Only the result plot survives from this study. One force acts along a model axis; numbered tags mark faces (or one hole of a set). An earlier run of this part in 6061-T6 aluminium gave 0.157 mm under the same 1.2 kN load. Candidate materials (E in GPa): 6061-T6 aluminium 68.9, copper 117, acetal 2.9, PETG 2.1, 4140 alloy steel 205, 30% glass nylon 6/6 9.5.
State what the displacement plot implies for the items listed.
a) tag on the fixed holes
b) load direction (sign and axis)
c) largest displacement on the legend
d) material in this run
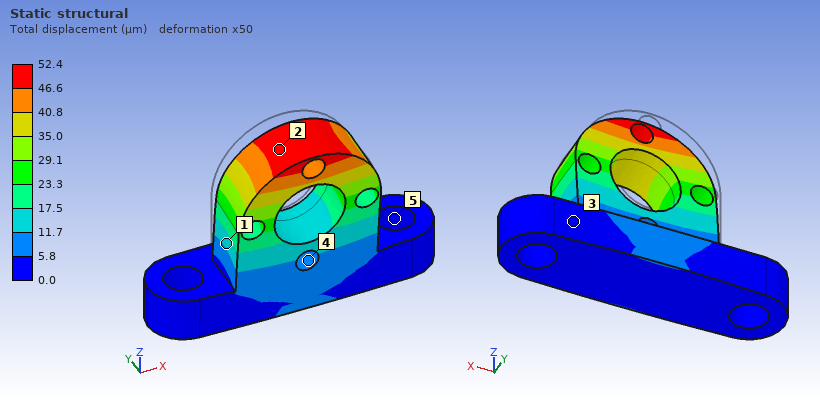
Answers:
5
-Y
52.4 µm
4140 alloy steel
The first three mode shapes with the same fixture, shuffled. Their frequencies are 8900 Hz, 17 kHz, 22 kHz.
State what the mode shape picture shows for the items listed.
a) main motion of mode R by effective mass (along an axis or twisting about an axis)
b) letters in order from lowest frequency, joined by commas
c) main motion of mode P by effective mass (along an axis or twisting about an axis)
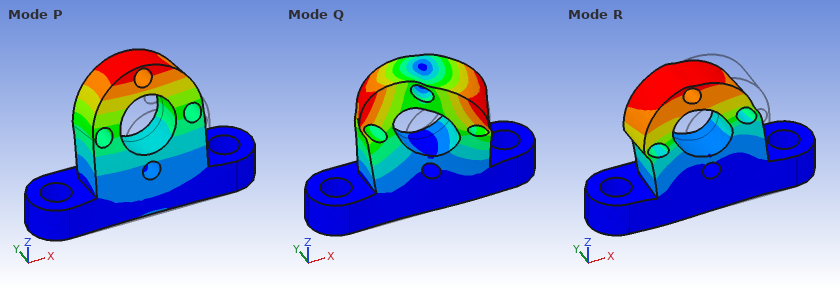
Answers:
along X
P, R, Q
along Y
